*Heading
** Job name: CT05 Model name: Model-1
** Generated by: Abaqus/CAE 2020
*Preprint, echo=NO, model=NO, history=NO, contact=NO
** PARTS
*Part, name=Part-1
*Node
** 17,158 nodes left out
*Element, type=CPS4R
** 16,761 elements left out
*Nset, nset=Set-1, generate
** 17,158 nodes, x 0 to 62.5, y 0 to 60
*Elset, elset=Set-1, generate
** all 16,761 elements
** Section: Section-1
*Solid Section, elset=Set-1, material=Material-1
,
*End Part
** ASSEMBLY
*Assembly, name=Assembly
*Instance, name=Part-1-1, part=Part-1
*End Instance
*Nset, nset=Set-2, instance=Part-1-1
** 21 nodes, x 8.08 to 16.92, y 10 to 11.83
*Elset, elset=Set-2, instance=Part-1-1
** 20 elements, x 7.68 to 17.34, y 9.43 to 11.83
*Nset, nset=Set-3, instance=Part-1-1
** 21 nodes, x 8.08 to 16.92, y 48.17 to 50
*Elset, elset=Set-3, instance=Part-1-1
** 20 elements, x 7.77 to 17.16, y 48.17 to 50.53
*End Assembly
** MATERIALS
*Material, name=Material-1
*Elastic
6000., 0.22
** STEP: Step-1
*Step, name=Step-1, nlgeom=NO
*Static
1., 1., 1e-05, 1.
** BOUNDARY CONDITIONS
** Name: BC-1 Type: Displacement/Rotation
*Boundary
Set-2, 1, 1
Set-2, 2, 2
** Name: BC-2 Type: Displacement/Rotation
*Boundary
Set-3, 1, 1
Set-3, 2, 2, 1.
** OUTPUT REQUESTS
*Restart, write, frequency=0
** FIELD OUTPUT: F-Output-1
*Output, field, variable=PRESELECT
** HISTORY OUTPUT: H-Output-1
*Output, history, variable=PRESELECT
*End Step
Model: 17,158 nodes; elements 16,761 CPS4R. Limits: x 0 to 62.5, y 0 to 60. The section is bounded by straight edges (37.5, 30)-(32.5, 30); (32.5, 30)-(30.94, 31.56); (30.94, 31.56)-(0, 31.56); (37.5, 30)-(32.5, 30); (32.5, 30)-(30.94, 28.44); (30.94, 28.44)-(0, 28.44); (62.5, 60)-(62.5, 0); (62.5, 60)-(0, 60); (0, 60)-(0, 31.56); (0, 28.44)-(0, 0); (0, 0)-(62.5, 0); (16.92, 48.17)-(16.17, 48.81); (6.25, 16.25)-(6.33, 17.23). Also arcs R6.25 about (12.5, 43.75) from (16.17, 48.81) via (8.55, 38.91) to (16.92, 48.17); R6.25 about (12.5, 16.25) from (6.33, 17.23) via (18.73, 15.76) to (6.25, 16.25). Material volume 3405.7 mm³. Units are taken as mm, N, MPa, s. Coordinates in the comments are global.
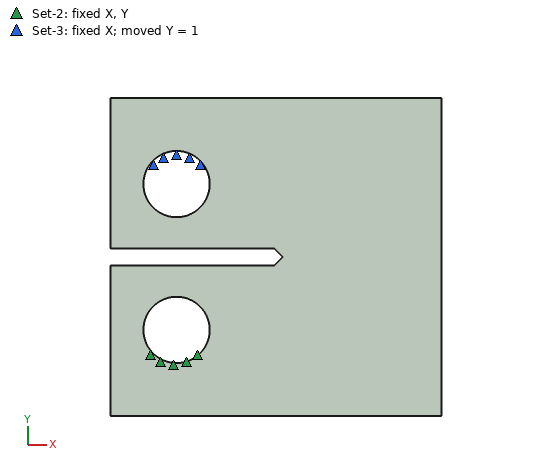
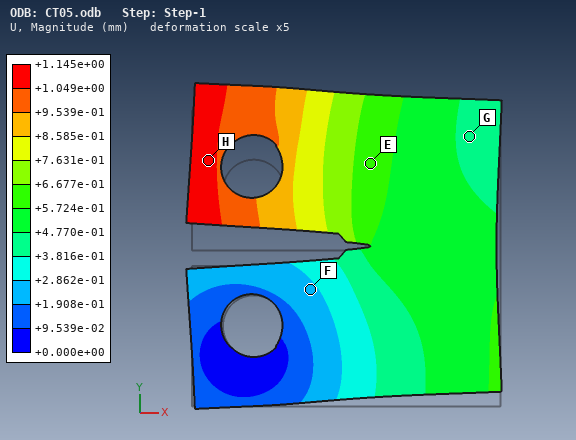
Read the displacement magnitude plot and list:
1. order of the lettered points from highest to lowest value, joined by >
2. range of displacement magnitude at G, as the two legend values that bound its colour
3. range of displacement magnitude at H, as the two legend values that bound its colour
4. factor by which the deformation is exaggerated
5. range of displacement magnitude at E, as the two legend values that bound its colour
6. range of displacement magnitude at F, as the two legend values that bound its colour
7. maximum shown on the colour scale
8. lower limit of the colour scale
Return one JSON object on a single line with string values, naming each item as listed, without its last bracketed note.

{"order of the lettered points from highest to lowest value, joined by >": "H > E > G > F", "range of displacement magnitude at G, as the two legend values that bound its colour": "+3.816e-01 to +4.770e-01 mm", "range of displacement magnitude at H, as the two legend values that bound its colour": "+1.049e+00 to +1.145e+00 mm", "factor by which the deformation is exaggerated": "5", "range of displacement magnitude at E, as the two legend values that bound its colour": "+5.724e-01 to +6.677e-01 mm", "range of displacement magnitude at F, as the two legend values that bound its colour": "+1.908e-01 to +2.862e-01 mm", "maximum shown on the colour scale": "+1.145e+00 mm", "lower limit of the colour scale": "+0.000e+00 mm"}
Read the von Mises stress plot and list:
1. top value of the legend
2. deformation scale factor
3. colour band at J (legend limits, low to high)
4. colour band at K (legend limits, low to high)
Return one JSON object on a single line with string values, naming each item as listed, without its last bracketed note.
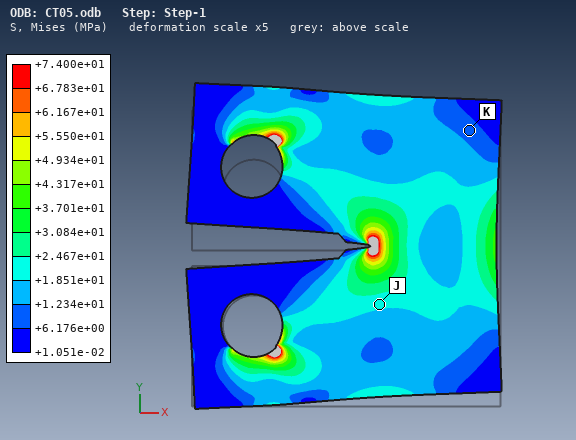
{"top value of the legend": "+7.400e+01 MPa", "deformation scale factor": "5", "colour band at J": "+1.851e+01 to +2.467e+01 MPa", "colour band at K": "+6.176e+00 to +1.234e+01 MPa"}
